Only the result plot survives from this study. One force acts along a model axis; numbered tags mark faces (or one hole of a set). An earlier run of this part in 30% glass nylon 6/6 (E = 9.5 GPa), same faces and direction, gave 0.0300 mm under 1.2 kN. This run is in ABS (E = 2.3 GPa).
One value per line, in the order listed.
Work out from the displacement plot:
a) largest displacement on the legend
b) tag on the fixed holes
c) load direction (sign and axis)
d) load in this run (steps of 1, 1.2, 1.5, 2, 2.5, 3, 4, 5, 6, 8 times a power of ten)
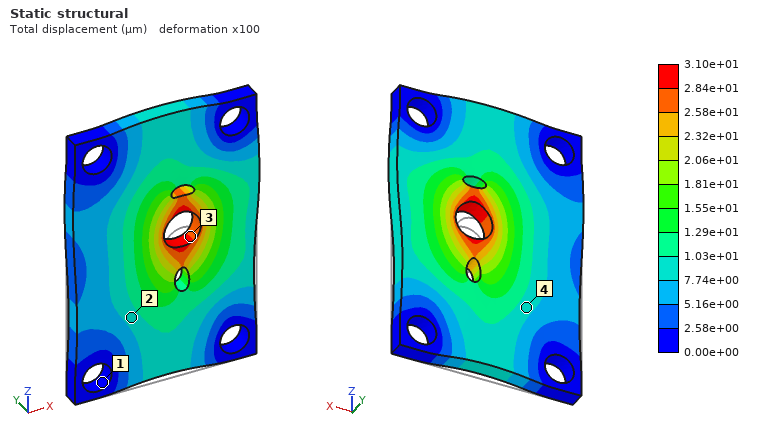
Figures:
3.10e+01 µm
1
+Z
300 N
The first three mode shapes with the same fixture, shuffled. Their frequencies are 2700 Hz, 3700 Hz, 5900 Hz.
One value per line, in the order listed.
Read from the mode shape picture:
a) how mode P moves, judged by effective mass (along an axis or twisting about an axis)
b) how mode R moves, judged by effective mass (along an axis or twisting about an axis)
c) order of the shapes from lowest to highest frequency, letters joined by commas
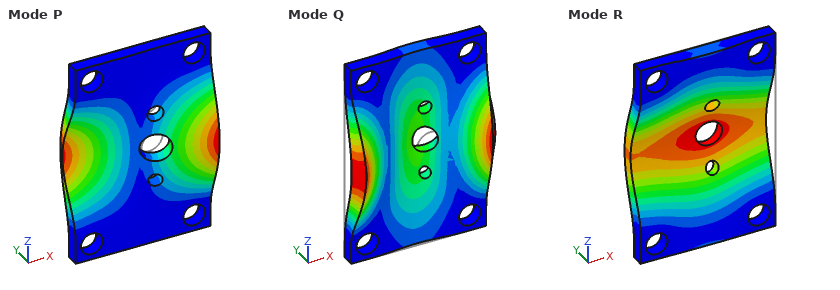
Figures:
twisting about Z
along Y
R, P, Q
